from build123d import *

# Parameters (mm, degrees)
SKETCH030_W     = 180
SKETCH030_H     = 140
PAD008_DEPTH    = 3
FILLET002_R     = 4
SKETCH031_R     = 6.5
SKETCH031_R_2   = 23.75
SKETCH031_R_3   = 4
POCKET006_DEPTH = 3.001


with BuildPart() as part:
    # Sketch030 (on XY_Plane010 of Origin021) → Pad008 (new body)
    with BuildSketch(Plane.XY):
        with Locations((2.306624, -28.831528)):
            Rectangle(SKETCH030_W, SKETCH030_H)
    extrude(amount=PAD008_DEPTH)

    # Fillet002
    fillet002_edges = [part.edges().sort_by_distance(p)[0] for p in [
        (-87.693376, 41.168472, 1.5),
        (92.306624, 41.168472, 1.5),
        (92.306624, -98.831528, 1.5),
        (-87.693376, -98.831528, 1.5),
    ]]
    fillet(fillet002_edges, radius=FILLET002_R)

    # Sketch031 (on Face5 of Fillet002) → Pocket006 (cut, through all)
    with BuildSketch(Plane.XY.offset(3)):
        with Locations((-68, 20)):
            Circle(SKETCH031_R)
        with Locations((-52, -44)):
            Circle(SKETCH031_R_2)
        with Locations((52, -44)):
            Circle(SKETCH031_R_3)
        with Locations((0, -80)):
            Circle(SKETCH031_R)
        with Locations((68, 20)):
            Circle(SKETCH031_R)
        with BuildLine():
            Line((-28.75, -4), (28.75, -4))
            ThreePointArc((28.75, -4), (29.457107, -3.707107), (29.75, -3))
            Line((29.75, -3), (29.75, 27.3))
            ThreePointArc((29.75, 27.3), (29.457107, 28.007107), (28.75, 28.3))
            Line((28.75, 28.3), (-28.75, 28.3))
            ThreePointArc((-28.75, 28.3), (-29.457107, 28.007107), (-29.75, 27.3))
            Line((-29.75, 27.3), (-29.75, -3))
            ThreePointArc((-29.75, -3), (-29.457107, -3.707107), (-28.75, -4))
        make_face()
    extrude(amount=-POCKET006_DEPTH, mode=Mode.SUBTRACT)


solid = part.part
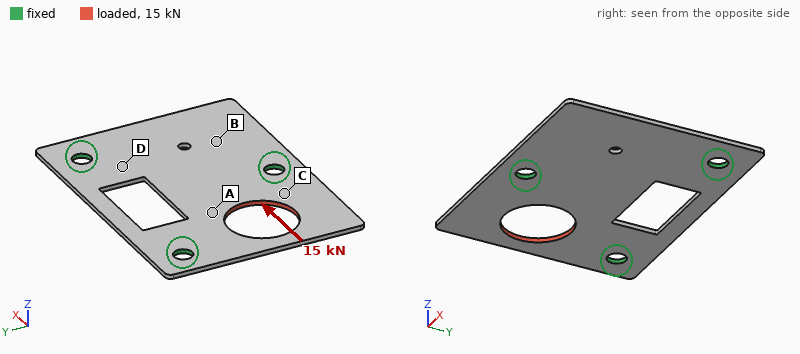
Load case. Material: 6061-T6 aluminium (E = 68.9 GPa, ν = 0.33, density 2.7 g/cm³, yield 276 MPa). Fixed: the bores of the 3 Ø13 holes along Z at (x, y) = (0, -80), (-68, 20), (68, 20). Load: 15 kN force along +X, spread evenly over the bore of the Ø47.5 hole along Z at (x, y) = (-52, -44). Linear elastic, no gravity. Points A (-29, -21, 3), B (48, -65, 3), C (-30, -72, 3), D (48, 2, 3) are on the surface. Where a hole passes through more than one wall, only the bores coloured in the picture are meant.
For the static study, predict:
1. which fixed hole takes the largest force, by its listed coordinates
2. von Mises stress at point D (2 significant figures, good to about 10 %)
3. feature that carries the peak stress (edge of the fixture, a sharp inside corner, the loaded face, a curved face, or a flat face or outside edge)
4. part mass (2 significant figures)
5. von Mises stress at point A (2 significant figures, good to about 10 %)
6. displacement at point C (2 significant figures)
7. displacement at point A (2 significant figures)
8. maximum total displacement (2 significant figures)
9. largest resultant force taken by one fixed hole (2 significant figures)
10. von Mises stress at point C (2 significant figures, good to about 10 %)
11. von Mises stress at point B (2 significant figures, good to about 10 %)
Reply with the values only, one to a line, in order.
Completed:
(0, -80)
30 MPa
a curved face
170 g
71 MPa
0.031 mm
0.067 mm
0.15 mm
9.2 kN
84 MPa
14 MPa
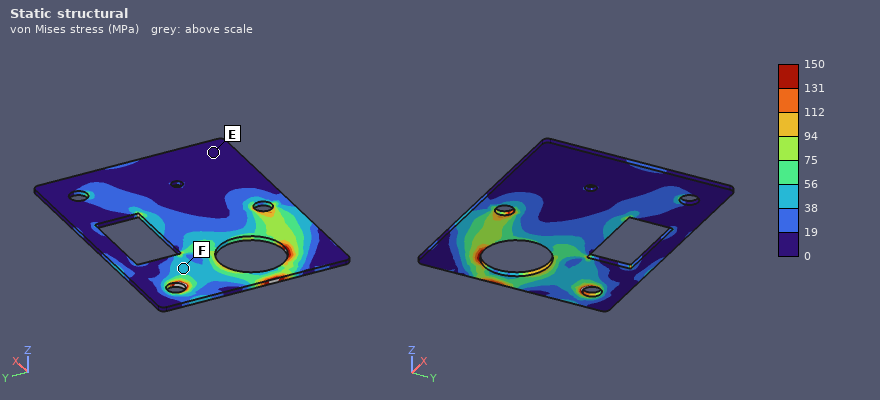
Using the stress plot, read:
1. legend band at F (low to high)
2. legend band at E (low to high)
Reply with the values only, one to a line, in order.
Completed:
38 to 56 MPa
0 to 19 MPa
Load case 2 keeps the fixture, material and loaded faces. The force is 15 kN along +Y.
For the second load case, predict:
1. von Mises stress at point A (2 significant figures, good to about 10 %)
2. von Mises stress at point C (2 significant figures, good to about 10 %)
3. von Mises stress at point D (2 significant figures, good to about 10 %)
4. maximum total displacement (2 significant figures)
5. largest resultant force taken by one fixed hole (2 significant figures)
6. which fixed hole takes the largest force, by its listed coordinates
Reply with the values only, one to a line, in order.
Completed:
23 MPa
45 MPa
20 MPa
0.11 mm
8.9 kN
(-68, 20)
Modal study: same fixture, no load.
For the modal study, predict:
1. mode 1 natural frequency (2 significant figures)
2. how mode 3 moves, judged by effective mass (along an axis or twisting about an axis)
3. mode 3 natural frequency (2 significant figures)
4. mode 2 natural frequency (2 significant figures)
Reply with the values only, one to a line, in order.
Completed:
490 Hz
along Z
1100 Hz
510 Hz
